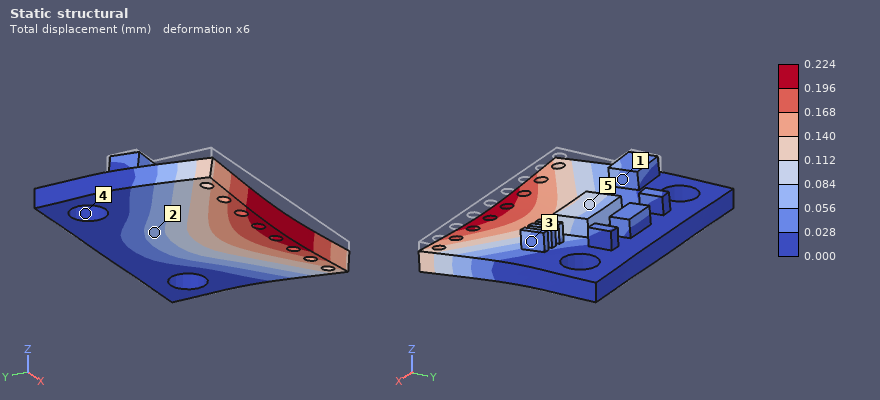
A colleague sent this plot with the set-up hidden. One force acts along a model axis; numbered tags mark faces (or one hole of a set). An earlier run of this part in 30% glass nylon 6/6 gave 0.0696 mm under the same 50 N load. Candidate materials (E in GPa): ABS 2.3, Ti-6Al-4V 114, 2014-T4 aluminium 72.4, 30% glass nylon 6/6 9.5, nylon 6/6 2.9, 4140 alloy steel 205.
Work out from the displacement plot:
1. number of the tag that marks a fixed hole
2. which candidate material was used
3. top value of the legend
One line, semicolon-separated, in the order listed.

4; nylon 6/6; 0.224 mm
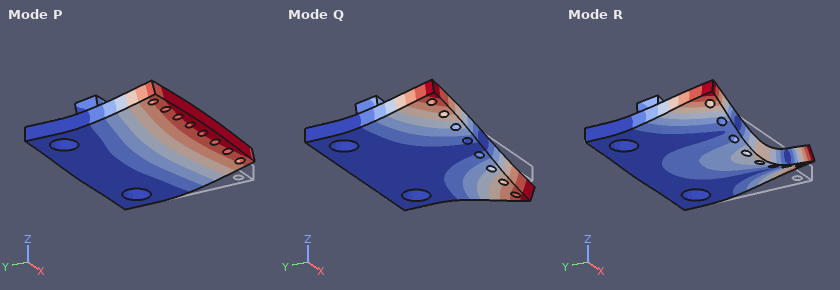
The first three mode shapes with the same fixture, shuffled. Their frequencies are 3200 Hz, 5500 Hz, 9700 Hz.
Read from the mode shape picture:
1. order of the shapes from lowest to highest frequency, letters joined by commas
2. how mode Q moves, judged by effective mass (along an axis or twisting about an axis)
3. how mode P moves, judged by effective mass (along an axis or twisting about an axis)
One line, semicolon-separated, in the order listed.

P, Q, R; twisting about Y; along Z
